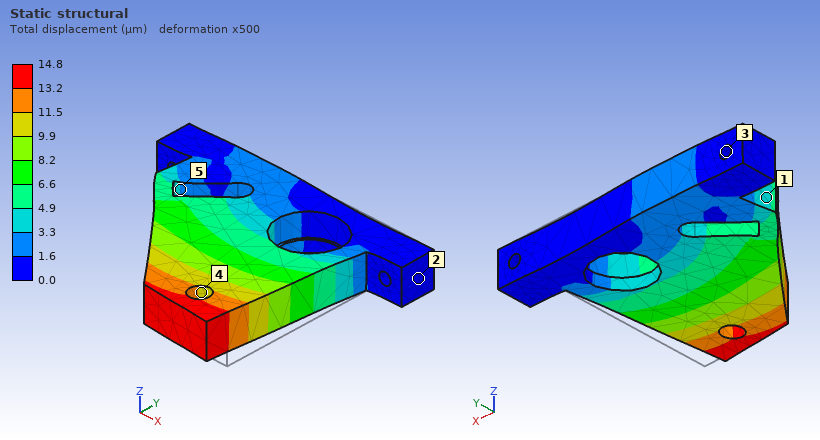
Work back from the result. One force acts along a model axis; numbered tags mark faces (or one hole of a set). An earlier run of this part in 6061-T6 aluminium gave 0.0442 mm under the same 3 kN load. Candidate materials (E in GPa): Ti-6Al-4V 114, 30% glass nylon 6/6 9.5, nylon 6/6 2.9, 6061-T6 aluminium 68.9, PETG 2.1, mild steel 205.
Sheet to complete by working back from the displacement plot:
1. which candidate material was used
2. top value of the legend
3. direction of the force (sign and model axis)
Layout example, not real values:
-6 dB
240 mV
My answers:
mild steel
14.8 µm
-X
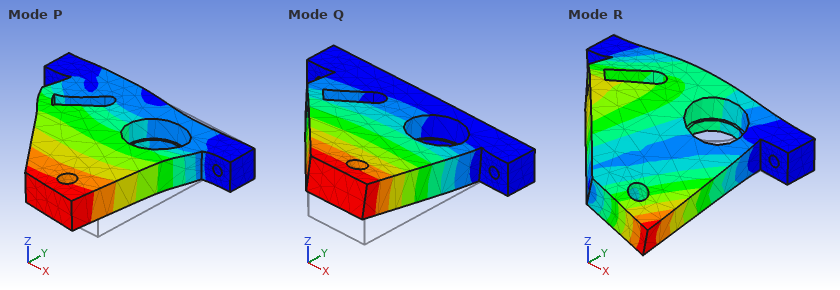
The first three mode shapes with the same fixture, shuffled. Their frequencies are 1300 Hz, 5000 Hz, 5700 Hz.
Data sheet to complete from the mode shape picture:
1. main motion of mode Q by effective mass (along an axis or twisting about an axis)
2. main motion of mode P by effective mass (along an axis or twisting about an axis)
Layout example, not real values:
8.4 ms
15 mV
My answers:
along Z
along X
